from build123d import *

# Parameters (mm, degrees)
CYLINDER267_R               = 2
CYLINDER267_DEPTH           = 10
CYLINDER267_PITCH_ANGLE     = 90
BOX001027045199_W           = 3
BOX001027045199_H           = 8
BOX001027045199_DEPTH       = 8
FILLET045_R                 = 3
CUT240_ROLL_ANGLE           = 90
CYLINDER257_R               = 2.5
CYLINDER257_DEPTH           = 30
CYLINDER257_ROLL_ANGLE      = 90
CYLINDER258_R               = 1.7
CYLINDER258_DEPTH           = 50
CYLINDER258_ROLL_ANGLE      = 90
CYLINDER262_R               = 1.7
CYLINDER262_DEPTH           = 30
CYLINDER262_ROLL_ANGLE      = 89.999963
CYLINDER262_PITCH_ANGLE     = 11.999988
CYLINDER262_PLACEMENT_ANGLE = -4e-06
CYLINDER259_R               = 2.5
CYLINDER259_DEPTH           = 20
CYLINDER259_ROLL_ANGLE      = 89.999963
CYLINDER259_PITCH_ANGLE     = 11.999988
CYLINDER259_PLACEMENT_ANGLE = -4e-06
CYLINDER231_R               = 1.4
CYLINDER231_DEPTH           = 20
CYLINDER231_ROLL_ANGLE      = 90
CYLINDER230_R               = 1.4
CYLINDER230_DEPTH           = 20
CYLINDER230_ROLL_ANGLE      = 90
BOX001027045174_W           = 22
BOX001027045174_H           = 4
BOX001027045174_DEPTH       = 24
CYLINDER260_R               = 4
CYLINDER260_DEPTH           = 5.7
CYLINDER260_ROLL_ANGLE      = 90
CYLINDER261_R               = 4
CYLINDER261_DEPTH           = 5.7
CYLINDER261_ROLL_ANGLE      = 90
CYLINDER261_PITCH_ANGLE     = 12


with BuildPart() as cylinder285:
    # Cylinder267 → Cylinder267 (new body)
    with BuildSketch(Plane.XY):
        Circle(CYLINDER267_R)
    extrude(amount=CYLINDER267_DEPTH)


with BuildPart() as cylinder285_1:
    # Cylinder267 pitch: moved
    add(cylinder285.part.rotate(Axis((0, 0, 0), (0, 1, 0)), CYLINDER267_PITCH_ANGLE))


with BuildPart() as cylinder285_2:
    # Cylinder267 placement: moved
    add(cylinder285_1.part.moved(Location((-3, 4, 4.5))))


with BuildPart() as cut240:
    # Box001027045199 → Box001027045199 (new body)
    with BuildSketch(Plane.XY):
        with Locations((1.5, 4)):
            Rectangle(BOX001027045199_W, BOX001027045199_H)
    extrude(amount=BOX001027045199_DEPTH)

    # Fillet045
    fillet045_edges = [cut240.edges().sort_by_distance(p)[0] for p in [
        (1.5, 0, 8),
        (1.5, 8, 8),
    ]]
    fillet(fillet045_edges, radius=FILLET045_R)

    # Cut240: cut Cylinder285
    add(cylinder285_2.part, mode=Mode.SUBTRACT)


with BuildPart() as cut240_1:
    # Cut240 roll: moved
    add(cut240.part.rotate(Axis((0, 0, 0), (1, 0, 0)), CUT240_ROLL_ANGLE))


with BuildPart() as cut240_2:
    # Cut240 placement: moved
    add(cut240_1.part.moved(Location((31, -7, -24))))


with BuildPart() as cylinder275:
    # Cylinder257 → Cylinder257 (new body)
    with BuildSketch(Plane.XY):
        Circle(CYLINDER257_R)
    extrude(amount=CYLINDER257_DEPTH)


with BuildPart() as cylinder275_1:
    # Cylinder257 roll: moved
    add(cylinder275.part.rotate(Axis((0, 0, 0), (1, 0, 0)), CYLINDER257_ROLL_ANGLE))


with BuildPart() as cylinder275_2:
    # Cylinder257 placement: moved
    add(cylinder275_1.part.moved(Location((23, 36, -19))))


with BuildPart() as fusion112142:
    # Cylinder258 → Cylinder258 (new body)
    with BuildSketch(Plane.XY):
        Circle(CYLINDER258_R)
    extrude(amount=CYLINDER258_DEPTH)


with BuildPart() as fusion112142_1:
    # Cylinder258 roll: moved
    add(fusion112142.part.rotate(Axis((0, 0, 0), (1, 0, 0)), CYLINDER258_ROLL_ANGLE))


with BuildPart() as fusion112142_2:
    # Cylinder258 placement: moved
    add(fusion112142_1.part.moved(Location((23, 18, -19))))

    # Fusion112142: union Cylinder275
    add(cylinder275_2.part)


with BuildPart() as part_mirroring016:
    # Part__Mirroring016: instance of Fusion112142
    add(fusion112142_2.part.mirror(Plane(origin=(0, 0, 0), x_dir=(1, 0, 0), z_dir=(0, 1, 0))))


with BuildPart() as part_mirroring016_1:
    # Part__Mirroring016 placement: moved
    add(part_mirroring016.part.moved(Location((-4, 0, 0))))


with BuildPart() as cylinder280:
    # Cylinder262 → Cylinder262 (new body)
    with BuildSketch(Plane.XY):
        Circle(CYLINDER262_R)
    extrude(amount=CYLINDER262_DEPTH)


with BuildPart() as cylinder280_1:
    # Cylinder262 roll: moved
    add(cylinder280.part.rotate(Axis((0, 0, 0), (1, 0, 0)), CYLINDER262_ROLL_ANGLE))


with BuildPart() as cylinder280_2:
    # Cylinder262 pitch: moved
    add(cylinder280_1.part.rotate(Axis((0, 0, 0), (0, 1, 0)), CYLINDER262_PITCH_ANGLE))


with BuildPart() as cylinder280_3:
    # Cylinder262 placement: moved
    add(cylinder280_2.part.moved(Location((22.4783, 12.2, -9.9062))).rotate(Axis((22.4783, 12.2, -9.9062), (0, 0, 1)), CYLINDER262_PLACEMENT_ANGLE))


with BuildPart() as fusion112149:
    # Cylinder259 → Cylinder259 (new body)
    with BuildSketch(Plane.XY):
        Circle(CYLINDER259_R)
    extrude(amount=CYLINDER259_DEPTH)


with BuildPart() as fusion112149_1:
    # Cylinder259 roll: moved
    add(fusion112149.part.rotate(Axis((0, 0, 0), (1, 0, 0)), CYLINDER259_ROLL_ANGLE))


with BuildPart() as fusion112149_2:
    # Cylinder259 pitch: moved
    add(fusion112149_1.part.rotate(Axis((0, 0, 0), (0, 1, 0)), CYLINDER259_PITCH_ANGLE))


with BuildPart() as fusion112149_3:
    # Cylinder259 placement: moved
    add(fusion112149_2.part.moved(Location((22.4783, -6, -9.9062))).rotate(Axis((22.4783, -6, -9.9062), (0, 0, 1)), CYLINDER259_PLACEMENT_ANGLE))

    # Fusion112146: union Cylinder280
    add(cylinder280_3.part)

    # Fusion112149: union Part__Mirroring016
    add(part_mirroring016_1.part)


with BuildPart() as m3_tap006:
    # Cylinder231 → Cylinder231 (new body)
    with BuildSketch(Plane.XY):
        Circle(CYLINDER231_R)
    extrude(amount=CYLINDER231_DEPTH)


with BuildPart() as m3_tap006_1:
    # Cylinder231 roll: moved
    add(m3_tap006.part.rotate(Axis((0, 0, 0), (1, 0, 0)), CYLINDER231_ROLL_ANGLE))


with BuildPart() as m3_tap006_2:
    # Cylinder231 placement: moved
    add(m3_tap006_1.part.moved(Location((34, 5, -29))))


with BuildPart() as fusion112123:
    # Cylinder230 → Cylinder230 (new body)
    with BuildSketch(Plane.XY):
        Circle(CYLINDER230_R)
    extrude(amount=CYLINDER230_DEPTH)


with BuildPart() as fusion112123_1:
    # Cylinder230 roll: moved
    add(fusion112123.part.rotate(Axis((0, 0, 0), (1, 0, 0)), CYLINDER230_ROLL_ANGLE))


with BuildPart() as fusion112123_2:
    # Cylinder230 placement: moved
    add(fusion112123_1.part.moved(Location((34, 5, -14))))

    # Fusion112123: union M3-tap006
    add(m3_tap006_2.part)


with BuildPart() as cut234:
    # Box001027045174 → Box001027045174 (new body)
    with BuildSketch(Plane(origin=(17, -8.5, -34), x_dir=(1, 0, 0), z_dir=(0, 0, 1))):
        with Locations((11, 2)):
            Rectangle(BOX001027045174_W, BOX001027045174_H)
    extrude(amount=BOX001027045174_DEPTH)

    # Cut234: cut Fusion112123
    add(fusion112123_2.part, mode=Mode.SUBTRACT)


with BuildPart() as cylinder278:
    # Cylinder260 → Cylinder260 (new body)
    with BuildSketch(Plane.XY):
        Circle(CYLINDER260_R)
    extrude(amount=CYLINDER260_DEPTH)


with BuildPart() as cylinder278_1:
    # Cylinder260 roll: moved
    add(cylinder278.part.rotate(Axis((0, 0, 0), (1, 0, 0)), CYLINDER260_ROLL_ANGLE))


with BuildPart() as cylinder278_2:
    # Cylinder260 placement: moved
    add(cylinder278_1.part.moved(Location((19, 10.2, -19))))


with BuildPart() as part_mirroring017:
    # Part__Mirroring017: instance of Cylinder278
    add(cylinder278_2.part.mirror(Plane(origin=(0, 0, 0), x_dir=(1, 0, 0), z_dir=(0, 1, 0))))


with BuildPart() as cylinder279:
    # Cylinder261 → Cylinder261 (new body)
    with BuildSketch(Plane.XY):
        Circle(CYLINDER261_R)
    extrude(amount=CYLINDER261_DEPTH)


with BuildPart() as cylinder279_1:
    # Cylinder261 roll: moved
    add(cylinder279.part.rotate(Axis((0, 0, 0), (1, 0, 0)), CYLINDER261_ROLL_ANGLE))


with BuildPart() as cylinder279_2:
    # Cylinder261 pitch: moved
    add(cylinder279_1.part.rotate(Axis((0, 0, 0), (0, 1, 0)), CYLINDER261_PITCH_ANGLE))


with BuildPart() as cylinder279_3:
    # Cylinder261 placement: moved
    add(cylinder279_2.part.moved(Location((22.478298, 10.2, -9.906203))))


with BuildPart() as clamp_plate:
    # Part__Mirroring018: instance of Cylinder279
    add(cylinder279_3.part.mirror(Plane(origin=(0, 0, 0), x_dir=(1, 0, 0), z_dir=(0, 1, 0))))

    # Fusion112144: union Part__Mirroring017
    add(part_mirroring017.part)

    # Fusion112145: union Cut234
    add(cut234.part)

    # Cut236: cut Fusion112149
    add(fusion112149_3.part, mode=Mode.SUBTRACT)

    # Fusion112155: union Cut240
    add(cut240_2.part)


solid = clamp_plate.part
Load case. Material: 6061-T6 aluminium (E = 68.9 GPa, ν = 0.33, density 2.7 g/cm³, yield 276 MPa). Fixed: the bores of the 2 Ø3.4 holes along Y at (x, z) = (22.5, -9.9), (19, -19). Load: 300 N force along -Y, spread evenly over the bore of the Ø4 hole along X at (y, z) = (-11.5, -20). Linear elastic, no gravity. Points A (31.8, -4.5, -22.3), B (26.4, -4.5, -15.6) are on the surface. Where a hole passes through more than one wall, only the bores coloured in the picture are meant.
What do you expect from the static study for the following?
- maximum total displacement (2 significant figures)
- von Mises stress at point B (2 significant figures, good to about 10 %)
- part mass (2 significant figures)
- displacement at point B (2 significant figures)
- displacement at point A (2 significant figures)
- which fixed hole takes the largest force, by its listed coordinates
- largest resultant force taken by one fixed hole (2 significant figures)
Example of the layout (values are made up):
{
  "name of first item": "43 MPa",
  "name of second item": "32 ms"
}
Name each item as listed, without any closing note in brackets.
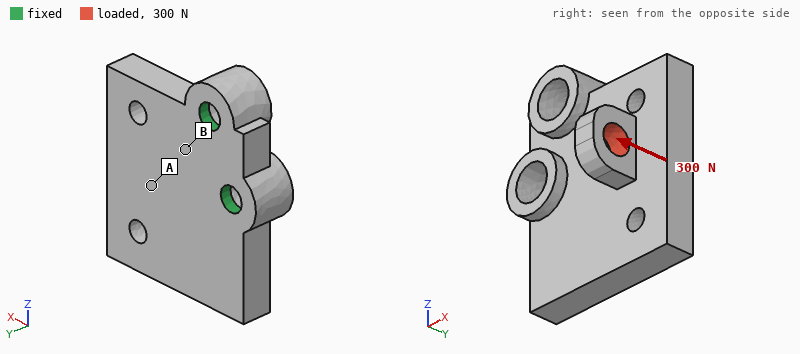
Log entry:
{
  "maximum total displacement": "0.13 mm",
  "von Mises stress at point B": "45 MPa",
  "part mass": "6.2 g",
  "displacement at point B": "0.022 mm",
  "displacement at point A": "0.066 mm",
  "which fixed hole takes the largest force, by its listed coordinates": "(19, -19)",
  "largest resultant force taken by one fixed hole": "190 N"
}
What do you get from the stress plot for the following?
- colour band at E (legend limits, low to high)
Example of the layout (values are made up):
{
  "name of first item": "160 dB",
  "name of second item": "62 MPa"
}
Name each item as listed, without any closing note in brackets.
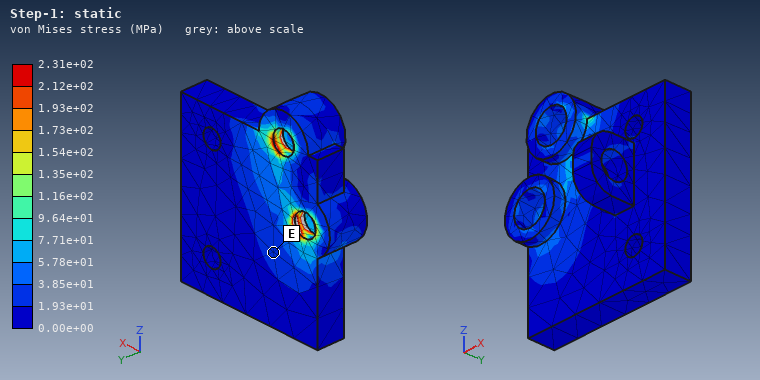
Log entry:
{
  "colour band at E": "1.93e+01 to 3.85e+01 MPa"
}
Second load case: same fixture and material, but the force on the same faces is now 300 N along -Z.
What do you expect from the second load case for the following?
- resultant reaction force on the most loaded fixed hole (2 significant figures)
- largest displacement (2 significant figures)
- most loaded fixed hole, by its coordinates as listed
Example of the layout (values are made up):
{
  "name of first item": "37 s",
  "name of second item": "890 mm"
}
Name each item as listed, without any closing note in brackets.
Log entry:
{
  "resultant reaction force on the most loaded fixed hole": "440 N",
  "largest displacement": "46 µm",
  "most loaded fixed hole, by its coordinates as listed": "(22.5, -9.9)"
}
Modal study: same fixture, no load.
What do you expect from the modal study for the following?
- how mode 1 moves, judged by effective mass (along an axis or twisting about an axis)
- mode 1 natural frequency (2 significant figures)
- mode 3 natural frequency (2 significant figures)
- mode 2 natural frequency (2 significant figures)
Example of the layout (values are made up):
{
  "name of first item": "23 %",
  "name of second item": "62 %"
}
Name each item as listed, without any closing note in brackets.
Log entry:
{
  "how mode 1 moves, judged by effective mass": "along Y",
  "mode 1 natural frequency": "4800 Hz",
  "mode 3 natural frequency": "14 kHz",
  "mode 2 natural frequency": "11 kHz"
}
